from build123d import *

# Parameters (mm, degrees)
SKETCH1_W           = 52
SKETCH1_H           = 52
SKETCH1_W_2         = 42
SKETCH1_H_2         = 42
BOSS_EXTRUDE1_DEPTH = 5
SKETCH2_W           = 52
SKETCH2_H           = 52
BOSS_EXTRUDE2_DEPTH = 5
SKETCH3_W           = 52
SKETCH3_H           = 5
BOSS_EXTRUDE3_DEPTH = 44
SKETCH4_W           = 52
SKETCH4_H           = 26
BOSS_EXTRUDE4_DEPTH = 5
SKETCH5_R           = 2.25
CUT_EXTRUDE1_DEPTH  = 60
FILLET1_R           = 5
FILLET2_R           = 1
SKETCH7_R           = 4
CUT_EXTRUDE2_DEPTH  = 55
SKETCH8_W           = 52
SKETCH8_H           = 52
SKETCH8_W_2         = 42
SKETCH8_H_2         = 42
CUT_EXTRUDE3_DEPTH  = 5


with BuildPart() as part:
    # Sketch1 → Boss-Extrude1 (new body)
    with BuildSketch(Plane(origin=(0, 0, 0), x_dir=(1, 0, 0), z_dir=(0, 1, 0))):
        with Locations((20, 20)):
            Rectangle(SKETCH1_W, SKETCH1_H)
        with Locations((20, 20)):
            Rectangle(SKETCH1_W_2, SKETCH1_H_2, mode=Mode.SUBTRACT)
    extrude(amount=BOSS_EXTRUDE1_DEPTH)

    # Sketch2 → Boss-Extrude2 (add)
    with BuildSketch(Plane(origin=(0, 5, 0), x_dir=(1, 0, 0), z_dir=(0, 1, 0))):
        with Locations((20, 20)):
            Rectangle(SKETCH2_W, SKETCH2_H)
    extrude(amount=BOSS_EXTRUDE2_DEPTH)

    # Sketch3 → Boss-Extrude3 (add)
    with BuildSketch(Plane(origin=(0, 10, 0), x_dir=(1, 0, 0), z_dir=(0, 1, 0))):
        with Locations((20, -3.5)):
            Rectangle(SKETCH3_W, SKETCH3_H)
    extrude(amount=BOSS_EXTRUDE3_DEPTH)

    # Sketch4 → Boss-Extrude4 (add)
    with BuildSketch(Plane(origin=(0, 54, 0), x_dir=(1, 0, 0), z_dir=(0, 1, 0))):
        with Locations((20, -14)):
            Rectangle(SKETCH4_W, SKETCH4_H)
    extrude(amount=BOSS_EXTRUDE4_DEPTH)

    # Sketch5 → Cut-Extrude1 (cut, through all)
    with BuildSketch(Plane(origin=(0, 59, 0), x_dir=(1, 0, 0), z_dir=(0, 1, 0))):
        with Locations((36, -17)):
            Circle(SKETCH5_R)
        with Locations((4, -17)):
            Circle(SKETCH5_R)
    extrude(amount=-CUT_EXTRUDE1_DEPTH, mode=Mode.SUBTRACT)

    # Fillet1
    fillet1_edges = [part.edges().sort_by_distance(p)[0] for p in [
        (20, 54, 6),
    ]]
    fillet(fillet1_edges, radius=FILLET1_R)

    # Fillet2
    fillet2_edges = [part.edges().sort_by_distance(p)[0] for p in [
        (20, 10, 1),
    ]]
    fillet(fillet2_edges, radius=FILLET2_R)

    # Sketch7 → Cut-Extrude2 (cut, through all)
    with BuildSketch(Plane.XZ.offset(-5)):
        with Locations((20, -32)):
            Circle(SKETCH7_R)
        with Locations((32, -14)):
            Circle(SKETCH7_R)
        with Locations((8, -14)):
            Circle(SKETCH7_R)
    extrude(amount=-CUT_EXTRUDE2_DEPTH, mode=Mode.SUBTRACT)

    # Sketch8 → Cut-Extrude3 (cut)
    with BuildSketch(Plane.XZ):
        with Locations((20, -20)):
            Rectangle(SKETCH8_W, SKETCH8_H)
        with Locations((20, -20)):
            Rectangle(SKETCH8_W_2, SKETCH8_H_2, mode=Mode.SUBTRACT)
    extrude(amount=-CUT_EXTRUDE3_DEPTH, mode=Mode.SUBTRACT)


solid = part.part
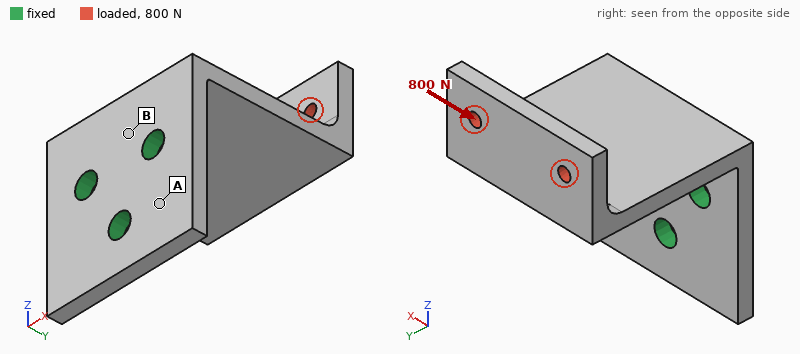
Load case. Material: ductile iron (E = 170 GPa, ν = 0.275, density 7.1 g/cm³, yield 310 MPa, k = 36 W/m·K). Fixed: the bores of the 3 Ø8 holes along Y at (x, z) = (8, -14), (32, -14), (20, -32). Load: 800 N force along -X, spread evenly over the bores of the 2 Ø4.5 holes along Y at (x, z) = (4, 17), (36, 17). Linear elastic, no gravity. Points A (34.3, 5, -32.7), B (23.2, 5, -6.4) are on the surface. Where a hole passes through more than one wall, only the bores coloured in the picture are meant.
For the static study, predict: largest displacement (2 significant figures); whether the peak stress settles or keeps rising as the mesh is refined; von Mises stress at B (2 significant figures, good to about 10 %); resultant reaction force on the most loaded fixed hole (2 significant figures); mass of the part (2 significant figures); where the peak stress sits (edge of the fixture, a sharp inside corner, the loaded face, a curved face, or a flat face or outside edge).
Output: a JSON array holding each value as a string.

["0.11 mm", "keeps rising", "31 MPa", "1.5 kN", "220 g", "edge of the fixture"]
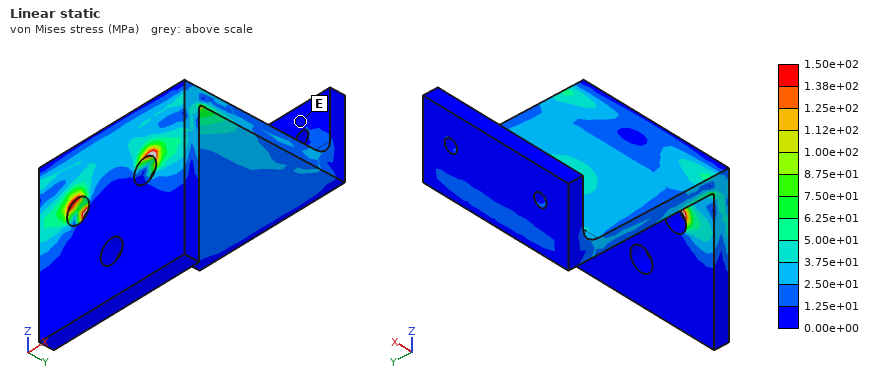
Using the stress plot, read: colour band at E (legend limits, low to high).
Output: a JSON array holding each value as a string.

["0.00e+00 to 1.25e+01 MPa"]
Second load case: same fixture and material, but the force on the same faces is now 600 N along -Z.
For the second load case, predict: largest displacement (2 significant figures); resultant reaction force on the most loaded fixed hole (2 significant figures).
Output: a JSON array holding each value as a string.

["0.57 mm", "310 N"]
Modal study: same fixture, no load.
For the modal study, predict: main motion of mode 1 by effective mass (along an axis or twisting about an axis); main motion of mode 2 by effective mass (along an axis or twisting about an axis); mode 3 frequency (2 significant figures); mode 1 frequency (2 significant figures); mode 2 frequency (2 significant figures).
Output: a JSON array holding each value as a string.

["along Z", "along X", "2100 Hz", "660 Hz", "1900 Hz"]
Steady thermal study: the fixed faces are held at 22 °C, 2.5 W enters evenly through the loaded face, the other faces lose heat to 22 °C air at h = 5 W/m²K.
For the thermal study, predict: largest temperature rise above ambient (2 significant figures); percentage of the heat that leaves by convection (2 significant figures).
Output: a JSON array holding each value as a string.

["18 K", "19 %"]
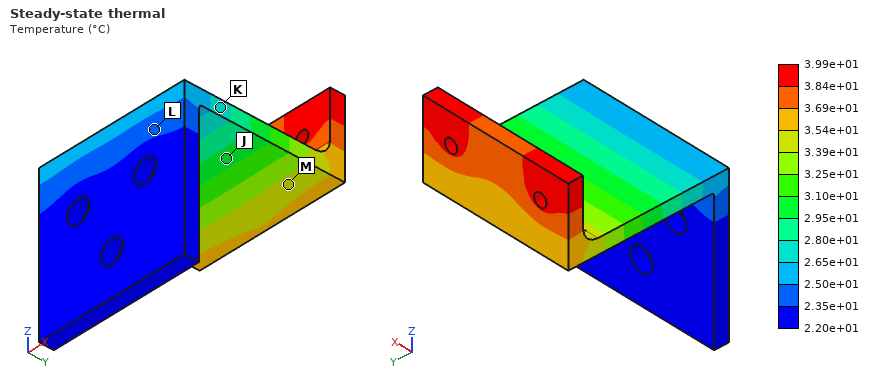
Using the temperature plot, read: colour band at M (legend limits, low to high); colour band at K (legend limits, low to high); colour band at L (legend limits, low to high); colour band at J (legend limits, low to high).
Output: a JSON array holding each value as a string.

["3.39e+01 to 3.54e+01 °C", "2.65e+01 to 2.80e+01 °C", "2.35e+01 to 2.50e+01 °C", "2.95e+01 to 3.10e+01 °C"]
